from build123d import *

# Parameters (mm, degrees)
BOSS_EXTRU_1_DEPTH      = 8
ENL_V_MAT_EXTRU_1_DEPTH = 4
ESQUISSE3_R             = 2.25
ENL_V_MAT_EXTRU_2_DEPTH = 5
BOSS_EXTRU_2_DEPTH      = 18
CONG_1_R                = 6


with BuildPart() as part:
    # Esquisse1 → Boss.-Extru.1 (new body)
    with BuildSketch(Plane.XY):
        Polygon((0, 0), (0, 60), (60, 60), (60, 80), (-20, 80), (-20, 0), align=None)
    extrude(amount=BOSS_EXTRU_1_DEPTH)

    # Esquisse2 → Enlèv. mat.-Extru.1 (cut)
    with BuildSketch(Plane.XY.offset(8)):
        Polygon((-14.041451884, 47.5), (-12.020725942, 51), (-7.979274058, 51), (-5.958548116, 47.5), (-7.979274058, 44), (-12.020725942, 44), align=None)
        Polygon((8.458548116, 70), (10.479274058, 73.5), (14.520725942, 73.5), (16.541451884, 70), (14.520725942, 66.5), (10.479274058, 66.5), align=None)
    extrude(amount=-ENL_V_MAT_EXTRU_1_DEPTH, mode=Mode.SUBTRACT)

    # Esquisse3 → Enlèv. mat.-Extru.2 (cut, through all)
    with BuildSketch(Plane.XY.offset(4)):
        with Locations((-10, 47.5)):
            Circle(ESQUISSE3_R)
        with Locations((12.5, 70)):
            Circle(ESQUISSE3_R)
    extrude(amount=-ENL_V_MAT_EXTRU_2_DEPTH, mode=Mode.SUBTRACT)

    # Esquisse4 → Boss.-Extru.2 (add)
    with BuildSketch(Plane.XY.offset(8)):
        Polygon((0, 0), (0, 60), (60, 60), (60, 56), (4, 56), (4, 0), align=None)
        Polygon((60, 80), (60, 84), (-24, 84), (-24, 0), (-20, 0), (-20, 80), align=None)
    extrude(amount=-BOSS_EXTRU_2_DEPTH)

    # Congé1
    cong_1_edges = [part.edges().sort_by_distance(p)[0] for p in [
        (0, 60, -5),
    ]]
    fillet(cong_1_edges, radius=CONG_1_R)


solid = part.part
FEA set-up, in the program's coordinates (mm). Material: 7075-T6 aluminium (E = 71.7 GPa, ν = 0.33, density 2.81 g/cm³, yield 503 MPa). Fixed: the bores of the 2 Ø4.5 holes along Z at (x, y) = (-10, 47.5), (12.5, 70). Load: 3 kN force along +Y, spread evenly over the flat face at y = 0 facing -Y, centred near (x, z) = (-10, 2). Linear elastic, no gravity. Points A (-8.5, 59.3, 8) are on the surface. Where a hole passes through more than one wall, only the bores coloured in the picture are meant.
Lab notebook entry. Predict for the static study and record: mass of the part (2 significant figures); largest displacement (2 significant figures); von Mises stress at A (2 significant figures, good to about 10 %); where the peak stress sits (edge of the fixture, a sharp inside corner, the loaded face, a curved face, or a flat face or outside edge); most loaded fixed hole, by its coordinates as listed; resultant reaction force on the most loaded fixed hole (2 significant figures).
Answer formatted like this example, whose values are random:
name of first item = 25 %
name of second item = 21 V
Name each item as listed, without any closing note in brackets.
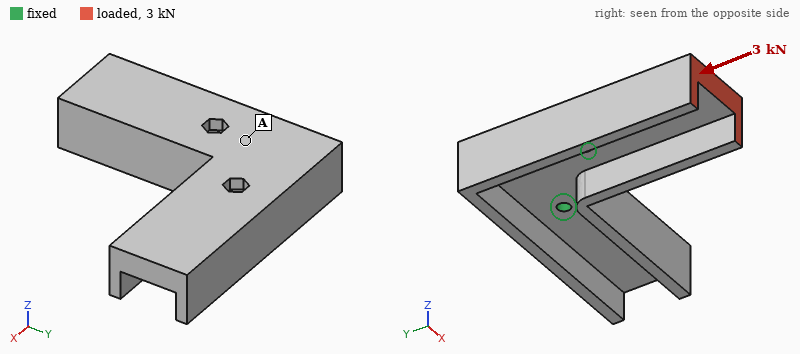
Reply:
mass of the part = 120 g
largest displacement = 15 µm
von Mises stress at A = 5.0 MPa
where the peak stress sits = edge of the fixture
most loaded fixed hole, by its coordinates as listed = (-10, 47.5)
resultant reaction force on the most loaded fixed hole = 2.7 kN
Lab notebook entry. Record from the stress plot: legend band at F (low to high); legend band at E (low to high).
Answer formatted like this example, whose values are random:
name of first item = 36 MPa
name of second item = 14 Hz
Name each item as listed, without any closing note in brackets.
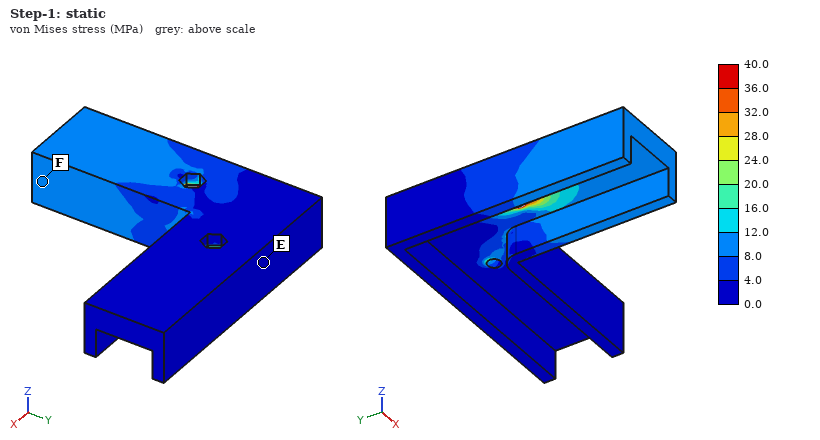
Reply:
legend band at F = 8.0 to 12.0 MPa
legend band at E = 0.0 to 4.0 MPa
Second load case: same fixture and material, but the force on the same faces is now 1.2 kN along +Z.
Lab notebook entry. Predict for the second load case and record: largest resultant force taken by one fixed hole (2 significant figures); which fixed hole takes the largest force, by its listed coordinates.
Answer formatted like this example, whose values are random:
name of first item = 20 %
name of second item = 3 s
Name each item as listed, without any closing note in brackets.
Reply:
largest resultant force taken by one fixed hole = 2.4 kN
which fixed hole takes the largest force, by its listed coordinates = (-10, 47.5)
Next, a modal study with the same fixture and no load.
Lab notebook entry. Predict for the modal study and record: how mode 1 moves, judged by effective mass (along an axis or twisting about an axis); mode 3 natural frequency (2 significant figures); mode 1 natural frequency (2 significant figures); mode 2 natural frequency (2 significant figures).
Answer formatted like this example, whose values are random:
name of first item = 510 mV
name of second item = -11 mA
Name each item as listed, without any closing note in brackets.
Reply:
how mode 1 moves, judged by effective mass = along Z
mode 3 natural frequency = 4700 Hz
mode 1 natural frequency = 2000 Hz
mode 2 natural frequency = 3300 Hz
